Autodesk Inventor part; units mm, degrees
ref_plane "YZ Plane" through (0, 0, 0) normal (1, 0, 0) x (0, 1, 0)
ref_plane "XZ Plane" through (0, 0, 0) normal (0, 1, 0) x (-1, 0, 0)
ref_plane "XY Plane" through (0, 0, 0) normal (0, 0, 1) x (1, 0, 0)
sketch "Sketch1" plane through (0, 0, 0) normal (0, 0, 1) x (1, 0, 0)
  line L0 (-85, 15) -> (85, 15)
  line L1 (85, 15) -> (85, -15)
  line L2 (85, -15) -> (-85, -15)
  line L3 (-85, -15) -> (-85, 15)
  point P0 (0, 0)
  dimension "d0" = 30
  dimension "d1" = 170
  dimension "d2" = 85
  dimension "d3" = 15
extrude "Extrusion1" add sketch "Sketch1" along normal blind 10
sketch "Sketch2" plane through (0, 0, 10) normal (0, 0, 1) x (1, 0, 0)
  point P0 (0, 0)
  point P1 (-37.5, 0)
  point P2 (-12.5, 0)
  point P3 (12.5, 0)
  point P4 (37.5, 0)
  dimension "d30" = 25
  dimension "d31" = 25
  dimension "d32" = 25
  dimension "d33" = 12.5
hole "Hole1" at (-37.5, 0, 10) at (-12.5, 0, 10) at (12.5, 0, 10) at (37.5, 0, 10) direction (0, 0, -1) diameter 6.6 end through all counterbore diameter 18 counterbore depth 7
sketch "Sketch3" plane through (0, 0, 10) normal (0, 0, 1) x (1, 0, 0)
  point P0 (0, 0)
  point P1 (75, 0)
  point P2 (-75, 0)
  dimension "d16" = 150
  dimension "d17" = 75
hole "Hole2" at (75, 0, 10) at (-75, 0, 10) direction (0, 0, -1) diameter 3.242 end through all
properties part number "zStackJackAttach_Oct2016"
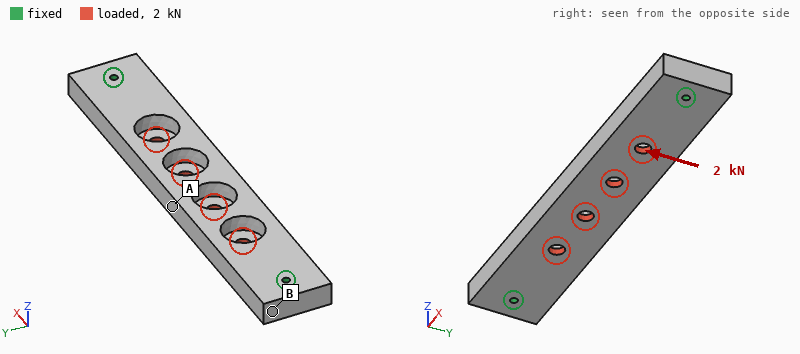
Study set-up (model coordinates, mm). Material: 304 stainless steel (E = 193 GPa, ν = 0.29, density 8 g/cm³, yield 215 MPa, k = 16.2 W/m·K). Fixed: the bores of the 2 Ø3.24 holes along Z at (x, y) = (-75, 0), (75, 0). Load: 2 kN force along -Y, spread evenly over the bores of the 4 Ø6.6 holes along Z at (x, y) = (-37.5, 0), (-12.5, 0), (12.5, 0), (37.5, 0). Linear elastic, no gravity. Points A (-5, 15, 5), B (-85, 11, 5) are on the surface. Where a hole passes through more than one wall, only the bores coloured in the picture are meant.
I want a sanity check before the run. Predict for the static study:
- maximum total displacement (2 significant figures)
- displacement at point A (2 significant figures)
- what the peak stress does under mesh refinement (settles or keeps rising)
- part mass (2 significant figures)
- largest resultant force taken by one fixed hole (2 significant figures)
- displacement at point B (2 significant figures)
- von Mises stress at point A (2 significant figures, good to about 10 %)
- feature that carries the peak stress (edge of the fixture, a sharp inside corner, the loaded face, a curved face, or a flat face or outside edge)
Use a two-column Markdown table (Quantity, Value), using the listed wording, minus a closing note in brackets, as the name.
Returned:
| Quantity | Value |
|---|---|
| maximum total displacement | 28 µm |
| displacement at point A | 26 µm |
| what the peak stress does under mesh refinement | keeps rising |
| part mass | 350 g |
| largest resultant force taken by one fixed hole | 1.0 kN |
| displacement at point B | 6.2 µm |
| von Mises stress at point A | 32 MPa |
| feature that carries the peak stress | edge of the fixture |
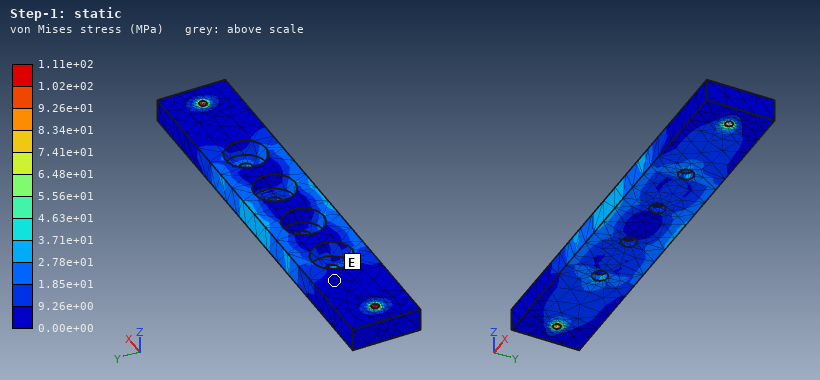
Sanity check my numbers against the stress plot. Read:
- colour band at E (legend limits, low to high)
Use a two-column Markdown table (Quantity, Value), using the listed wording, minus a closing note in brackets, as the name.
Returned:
| Quantity | Value |
|---|---|
| colour band at E | 0.00e+00 to 9.26e+00 MPa |
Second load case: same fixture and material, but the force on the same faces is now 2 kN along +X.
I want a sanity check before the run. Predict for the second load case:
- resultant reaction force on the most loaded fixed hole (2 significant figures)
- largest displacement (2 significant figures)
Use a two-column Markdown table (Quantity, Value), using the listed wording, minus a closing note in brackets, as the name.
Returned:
| Quantity | Value |
|---|---|
| resultant reaction force on the most loaded fixed hole | 1.0 kN |
| largest displacement | 1.8 µm |
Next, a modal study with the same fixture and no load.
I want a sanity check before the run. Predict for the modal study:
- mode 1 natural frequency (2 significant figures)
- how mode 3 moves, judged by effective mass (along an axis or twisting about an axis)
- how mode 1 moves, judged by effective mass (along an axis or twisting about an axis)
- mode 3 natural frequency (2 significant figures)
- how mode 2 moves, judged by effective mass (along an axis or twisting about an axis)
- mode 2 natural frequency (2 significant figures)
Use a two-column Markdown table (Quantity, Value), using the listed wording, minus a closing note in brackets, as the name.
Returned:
| Quantity | Value |
|---|---|
| mode 1 natural frequency | 2100 Hz |
| how mode 3 moves, judged by effective mass | twisting about X |
| how mode 1 moves, judged by effective mass | along Z |
| mode 3 natural frequency | 4900 Hz |
| how mode 2 moves, judged by effective mass | along Y |
| mode 2 natural frequency | 3400 Hz |
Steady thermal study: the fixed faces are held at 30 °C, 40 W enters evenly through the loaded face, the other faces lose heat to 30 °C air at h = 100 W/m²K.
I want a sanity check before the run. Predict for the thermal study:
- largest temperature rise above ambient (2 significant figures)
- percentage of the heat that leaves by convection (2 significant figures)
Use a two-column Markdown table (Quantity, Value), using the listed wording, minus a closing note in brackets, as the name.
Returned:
| Quantity | Value |
|---|---|
| largest temperature rise above ambient | 74 K |
| percentage of the heat that leaves by convection | 90 % |
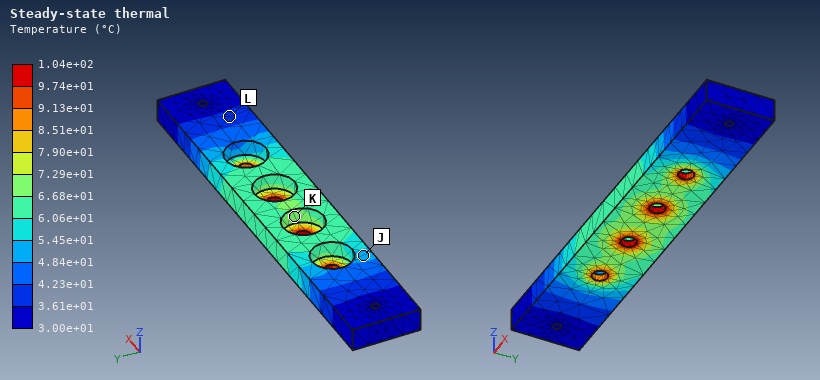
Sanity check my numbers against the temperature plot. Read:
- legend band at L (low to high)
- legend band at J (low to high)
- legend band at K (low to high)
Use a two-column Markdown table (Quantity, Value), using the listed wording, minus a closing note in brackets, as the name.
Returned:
| Quantity | Value |
|---|---|
| legend band at L | 3.61e+01 to 4.23e+01 °C |
| legend band at J | 4.84e+01 to 5.45e+01 °C |
| legend band at K | 6.68e+01 to 7.29e+01 °C |
